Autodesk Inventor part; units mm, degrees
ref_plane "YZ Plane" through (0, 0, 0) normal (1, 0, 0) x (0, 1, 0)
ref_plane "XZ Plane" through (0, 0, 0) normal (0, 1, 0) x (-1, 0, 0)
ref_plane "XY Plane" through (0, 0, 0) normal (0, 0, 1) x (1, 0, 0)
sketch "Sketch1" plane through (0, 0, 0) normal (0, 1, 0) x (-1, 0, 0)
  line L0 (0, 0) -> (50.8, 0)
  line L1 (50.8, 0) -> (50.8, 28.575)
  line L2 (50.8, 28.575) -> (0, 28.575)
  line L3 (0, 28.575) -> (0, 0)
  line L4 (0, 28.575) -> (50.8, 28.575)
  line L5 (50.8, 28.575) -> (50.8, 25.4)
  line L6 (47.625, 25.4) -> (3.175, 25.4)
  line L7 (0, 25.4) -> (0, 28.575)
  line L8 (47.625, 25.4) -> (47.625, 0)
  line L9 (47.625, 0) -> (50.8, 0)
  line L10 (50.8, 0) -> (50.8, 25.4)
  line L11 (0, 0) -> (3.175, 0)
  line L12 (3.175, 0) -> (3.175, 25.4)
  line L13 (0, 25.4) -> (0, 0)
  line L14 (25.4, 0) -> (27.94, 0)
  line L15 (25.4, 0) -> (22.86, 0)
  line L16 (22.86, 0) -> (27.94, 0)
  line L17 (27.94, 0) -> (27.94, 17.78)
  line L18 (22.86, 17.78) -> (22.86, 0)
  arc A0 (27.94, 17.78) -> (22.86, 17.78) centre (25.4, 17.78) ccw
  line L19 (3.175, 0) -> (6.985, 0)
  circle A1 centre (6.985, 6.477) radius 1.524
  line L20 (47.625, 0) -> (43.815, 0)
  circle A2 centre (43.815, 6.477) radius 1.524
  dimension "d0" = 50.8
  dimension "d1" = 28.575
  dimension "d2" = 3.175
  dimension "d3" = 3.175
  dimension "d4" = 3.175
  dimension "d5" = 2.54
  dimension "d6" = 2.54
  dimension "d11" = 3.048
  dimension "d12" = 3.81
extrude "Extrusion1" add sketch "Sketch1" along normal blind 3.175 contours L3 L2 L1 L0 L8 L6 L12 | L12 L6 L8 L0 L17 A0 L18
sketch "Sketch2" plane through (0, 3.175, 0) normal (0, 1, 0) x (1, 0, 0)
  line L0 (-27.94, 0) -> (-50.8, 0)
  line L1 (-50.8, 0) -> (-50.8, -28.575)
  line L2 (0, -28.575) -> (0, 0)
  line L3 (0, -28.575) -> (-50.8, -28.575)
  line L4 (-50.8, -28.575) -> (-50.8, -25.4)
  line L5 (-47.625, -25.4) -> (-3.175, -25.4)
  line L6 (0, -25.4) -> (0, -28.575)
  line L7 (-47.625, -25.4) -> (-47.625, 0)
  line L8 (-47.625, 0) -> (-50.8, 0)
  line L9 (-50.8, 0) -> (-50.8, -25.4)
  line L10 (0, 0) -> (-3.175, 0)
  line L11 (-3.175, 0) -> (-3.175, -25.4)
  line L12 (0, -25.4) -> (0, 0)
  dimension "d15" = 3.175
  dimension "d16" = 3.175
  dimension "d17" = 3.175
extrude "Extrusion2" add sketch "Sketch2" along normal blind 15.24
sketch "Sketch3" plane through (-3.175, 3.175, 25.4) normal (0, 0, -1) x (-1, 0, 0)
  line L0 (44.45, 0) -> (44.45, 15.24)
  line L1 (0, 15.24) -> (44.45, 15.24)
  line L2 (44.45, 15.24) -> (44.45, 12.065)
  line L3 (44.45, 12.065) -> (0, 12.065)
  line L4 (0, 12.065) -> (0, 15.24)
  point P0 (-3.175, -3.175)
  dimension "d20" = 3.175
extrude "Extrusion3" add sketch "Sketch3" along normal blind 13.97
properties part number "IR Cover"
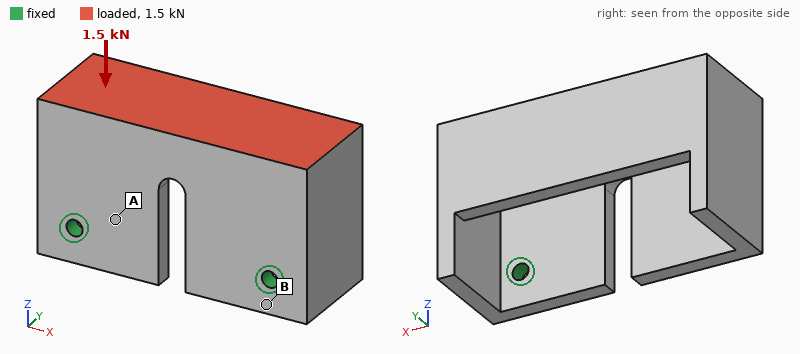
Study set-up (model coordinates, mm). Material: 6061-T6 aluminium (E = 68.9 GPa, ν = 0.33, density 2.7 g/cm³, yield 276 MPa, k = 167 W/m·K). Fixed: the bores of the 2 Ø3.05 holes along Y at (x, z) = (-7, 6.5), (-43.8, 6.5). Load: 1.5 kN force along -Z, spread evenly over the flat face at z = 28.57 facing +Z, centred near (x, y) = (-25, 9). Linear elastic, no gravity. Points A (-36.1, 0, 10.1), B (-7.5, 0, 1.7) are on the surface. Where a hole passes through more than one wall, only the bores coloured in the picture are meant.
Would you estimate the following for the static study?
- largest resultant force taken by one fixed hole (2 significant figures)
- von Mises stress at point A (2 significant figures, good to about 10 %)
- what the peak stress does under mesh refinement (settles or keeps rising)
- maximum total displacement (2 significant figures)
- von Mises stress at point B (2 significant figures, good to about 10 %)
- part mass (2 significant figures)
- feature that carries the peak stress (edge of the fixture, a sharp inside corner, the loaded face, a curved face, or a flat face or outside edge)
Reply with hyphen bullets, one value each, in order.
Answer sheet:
- 750 N
- 32 MPa
- keeps rising
- 0.15 mm
- 78 MPa
- 30 g
- edge of the fixture
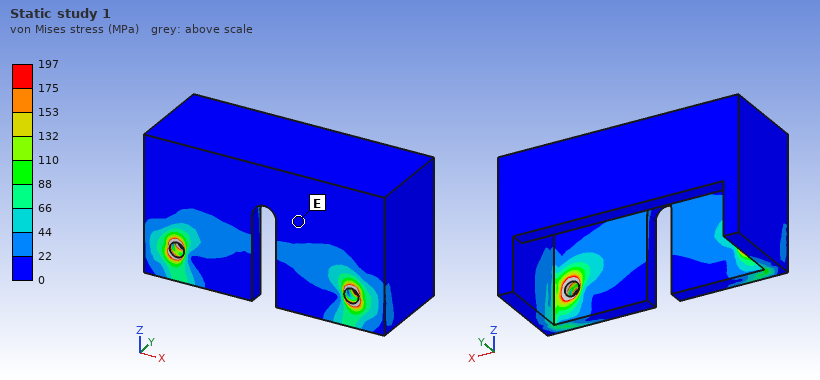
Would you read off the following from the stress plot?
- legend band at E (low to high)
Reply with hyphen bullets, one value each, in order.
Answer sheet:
- 0 to 22 MPa
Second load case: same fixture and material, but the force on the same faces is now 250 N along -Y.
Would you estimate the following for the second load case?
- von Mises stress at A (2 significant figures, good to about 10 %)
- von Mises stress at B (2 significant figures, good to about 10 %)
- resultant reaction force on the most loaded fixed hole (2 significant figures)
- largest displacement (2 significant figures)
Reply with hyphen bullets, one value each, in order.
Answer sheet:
- 17 MPa
- 26 MPa
- 130 N
- 70 µm
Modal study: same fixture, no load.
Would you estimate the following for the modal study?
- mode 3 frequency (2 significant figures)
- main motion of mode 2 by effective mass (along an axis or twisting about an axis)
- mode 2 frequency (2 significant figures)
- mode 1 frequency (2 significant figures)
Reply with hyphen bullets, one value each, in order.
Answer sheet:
- 9400 Hz
- along X
- 4000 Hz
- 2600 Hz
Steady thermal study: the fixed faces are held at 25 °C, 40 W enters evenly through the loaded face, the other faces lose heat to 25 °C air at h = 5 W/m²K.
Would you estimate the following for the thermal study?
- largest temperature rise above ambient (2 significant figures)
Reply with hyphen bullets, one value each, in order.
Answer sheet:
- 32 K
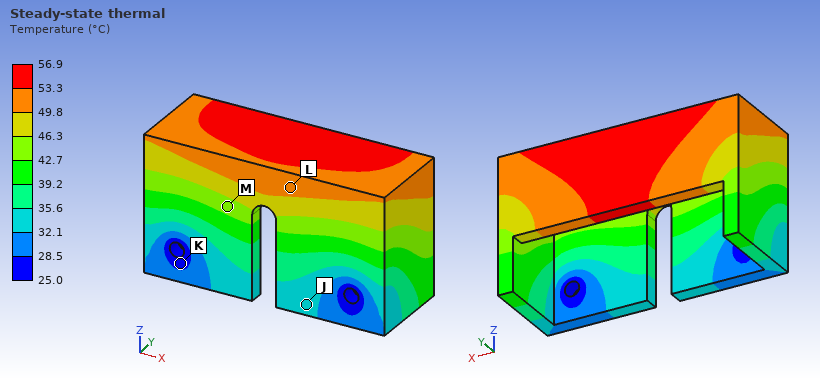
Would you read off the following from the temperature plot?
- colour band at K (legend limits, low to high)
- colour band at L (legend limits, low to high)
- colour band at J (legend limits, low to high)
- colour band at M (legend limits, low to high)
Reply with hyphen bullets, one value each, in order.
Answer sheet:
- 25.0 to 28.5 °C
- 49.8 to 53.3 °C
- 32.1 to 35.6 °C
- 42.7 to 46.3 °C
